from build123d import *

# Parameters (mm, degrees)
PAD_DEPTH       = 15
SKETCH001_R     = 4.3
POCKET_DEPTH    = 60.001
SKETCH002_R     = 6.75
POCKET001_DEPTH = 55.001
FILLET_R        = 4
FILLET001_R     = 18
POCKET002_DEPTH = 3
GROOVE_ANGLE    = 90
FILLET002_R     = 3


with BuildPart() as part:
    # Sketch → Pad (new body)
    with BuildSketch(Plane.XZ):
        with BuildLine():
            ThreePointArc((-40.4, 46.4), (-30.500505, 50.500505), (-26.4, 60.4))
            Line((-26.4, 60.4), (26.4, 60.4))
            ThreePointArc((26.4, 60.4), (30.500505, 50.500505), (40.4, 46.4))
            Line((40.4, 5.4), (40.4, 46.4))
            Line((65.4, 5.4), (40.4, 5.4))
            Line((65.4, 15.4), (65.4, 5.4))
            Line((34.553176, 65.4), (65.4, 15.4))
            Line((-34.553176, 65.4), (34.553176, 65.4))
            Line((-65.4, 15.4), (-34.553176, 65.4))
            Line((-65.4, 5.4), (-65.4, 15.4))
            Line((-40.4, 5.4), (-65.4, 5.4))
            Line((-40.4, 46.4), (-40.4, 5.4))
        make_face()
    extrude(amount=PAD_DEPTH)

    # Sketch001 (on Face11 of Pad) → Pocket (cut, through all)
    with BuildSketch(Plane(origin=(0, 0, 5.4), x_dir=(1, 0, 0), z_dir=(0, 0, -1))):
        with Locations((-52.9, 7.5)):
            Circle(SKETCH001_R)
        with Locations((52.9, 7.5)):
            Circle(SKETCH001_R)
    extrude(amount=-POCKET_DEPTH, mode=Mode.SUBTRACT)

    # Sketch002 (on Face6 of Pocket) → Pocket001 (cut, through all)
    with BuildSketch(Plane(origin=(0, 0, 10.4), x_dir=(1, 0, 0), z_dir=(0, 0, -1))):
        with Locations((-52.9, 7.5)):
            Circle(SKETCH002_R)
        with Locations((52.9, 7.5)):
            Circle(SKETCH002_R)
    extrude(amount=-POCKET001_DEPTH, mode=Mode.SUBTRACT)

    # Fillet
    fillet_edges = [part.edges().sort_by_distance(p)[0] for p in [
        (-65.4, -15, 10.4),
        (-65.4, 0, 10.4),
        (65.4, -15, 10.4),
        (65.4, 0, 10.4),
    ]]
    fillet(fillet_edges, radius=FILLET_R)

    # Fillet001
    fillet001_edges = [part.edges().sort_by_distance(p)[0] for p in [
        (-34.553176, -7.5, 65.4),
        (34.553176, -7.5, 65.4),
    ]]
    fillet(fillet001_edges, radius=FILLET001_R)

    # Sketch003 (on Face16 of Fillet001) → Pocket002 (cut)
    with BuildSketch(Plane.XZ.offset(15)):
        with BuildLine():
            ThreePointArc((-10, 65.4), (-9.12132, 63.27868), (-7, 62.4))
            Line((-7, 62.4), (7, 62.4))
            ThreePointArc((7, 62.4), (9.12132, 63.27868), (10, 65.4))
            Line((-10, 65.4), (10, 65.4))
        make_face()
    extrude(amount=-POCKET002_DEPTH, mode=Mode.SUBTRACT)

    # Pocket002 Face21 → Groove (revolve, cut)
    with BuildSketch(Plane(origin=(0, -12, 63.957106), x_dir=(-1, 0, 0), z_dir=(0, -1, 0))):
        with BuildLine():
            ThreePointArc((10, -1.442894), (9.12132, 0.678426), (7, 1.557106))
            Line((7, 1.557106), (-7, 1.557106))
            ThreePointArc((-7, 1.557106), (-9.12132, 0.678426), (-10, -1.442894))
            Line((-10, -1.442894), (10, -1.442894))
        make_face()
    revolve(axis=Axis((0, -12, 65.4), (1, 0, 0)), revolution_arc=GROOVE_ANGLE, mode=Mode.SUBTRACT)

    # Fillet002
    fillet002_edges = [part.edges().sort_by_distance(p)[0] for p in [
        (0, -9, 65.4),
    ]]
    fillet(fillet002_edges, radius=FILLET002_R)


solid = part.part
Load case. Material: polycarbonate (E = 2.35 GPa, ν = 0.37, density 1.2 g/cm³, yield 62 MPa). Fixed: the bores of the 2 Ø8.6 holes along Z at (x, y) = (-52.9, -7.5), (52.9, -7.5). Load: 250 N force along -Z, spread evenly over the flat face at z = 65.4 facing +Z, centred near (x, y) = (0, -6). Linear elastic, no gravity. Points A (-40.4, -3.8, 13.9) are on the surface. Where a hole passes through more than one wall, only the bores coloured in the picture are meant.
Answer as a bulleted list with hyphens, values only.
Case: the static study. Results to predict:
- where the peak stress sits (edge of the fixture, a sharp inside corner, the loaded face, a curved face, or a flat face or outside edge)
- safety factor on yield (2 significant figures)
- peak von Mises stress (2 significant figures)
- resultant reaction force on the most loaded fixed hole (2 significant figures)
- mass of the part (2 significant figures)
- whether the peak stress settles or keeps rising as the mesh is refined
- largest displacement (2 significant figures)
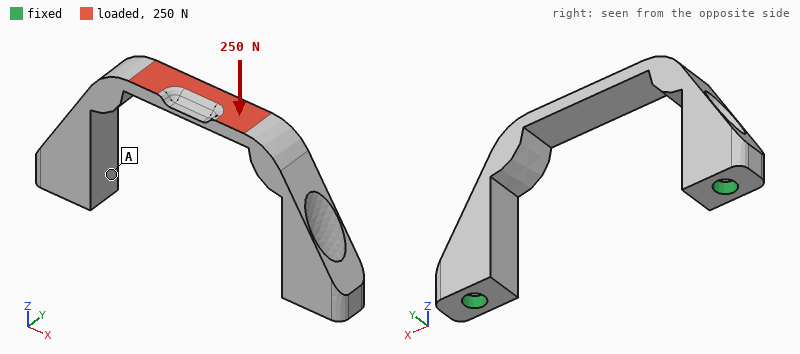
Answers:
- the loaded face
- 3.1
- 20 MPa
- 160 N
- 29 g
- settles
- 0.95 mm
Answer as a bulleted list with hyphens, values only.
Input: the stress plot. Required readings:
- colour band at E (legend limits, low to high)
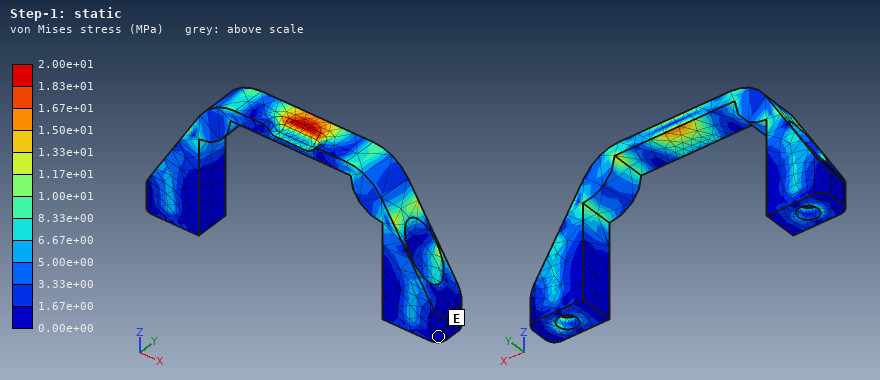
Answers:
- 0.00e+00 to 1.67e+00 MPa
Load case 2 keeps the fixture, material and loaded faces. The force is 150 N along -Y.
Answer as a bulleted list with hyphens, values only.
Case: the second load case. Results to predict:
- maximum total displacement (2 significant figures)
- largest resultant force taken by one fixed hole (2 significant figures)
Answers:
- 1.6 mm
- 75 N
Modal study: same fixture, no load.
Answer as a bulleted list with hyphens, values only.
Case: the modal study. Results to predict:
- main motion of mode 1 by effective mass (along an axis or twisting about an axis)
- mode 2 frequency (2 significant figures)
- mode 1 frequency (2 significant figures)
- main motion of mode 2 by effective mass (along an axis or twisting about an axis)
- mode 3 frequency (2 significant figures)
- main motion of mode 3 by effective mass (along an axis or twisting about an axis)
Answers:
- along Y
- 720 Hz
- 560 Hz
- along X
- 870 Hz
- twisting about Z
